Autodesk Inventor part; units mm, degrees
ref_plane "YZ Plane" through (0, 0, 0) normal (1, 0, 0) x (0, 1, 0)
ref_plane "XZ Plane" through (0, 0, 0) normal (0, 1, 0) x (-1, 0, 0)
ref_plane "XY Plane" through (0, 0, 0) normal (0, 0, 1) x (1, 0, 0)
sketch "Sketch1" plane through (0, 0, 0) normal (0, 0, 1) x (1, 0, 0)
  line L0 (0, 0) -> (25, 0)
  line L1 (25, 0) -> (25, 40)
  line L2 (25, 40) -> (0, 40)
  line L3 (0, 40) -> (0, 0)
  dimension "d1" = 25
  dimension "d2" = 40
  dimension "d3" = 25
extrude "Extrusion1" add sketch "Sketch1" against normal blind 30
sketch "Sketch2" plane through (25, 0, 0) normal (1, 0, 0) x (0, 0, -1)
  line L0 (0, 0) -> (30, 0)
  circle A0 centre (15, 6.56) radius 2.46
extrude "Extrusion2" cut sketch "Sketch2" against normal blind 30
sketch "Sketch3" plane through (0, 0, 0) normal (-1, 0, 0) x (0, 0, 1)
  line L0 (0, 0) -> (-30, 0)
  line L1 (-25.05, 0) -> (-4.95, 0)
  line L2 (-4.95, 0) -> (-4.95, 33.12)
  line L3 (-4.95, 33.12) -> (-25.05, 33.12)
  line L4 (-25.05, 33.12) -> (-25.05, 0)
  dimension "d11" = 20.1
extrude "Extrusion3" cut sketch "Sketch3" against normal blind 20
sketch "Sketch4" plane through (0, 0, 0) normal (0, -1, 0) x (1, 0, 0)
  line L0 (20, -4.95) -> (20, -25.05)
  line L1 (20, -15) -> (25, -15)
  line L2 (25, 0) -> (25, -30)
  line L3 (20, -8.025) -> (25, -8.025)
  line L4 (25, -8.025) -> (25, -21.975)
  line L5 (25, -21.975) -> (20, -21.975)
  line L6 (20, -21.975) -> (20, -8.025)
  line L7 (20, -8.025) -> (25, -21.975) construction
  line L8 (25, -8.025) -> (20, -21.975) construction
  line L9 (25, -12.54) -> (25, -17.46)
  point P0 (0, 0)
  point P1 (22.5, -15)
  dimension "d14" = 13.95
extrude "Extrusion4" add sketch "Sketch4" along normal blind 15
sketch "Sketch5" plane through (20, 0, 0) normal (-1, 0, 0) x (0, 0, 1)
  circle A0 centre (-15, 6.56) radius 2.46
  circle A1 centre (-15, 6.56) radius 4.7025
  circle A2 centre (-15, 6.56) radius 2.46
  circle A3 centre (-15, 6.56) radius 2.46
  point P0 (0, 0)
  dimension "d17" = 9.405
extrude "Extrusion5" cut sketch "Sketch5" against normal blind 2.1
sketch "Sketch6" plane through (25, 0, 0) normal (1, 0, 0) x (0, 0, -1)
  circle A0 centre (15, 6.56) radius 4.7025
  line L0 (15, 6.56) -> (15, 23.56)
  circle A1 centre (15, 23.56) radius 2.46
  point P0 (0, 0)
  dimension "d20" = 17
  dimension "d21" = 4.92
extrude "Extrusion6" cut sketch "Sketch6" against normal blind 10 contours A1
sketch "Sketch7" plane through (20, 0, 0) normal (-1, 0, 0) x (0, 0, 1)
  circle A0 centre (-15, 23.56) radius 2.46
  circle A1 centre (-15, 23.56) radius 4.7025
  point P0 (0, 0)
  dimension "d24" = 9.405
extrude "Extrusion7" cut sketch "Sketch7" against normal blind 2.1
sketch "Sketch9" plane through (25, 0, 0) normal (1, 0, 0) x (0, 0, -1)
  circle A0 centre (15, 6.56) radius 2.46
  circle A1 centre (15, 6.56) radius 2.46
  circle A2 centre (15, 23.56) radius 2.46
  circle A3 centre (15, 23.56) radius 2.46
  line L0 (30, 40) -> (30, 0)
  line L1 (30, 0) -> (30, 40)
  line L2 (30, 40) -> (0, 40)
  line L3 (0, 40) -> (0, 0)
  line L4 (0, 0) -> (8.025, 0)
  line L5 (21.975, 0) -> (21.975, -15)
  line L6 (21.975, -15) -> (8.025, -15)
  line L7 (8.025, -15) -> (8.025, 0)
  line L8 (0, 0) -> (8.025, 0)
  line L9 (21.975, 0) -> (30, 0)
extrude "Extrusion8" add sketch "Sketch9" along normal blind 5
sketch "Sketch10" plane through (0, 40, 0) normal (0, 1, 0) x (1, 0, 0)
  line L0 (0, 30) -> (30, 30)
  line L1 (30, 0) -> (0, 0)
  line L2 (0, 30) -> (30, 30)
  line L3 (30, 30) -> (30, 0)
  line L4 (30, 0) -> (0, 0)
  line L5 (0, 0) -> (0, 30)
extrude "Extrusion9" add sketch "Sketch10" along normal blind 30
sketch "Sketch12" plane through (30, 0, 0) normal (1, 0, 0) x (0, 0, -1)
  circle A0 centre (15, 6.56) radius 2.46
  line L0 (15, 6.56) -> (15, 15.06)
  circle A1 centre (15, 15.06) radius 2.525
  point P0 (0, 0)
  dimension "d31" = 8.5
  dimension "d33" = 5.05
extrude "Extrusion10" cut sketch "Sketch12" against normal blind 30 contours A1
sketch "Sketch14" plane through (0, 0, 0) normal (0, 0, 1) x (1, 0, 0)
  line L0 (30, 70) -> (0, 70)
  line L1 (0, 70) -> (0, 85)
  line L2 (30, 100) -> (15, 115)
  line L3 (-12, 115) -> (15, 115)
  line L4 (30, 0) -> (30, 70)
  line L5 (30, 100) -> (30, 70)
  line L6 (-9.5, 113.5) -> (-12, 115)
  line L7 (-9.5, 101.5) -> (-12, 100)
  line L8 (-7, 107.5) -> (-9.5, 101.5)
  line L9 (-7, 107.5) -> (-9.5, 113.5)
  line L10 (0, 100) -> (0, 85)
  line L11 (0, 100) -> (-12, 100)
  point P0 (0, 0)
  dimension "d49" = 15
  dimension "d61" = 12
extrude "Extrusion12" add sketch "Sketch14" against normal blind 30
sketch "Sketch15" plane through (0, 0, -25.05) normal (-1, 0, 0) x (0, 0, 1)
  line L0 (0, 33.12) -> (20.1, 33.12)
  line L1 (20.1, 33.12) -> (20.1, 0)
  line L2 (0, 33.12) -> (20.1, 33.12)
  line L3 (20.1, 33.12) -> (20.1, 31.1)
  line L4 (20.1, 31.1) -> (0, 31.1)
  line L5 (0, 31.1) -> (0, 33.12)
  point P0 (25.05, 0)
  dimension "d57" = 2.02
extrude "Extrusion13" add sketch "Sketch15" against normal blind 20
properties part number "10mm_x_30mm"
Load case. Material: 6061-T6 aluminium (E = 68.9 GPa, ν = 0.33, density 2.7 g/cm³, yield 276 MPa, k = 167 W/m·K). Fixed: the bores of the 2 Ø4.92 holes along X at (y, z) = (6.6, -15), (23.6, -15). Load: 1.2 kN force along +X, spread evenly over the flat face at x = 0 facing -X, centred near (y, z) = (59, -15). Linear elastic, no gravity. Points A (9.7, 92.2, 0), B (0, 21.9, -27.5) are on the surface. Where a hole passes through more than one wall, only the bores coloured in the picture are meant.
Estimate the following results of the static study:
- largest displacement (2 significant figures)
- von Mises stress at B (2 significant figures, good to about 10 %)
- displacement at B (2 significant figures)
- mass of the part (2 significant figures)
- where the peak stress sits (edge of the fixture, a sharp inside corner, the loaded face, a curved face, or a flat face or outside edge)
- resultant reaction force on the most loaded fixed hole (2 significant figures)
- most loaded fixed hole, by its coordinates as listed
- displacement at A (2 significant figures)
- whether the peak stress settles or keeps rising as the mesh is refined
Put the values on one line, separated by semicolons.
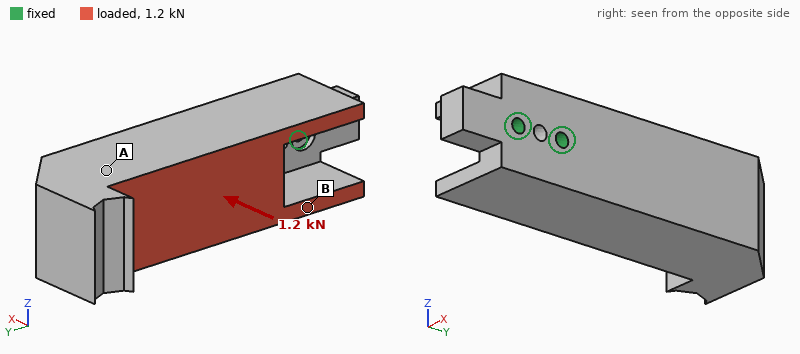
0.11 mm; 13 MPa; 0.022 mm; 250 g; edge of the fixture; 2.8 kN; (23.6, -15); 0.080 mm; keeps rising
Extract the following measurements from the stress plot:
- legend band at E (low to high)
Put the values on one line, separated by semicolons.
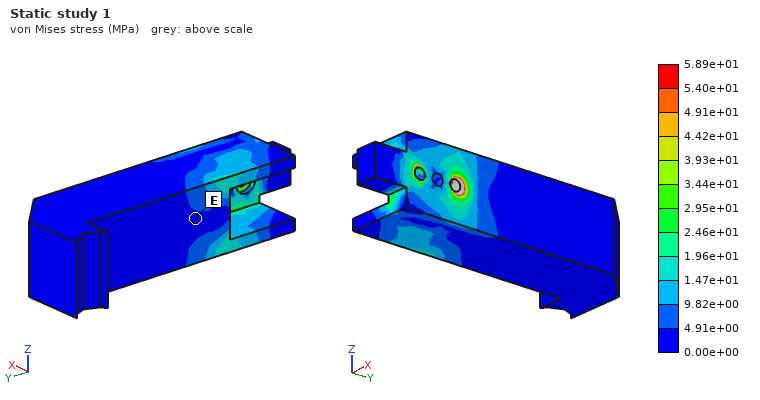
0.00e+00 to 4.91e+00 MPa
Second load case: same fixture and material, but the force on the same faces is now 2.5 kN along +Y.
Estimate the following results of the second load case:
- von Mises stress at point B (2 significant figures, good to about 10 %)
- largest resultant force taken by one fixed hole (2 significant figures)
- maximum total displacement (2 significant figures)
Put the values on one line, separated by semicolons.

17 MPa; 2.9 kN; 0.15 mm
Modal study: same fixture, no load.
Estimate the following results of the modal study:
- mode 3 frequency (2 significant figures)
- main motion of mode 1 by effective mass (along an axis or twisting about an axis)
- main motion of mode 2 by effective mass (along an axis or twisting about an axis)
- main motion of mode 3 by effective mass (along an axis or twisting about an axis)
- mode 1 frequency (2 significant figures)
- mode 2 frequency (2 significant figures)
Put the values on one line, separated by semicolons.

3400 Hz; along X; along Z; twisting about Y; 1200 Hz; 1400 Hz
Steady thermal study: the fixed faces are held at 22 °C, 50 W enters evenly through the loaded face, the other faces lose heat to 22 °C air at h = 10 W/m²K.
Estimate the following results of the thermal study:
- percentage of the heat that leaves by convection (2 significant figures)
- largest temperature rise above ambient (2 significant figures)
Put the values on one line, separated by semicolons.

4.2 %; 21 K
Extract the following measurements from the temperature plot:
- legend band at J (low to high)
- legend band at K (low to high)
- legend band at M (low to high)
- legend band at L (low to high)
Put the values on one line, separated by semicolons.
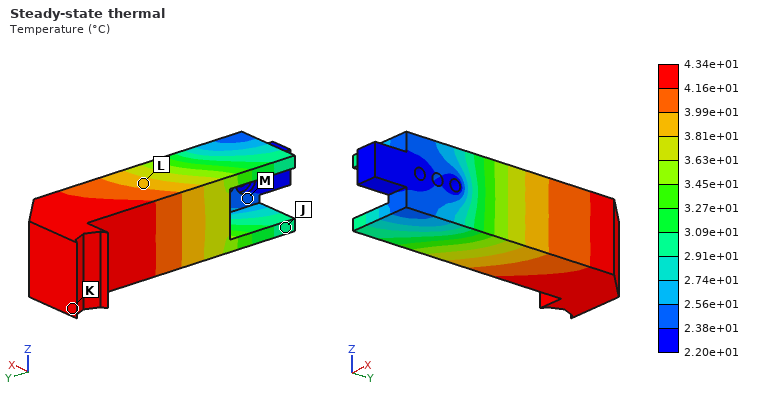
2.91e+01 to 3.09e+01 °C; 4.16e+01 to 4.34e+01 °C; 2.38e+01 to 2.56e+01 °C; 3.81e+01 to 3.99e+01 °C
